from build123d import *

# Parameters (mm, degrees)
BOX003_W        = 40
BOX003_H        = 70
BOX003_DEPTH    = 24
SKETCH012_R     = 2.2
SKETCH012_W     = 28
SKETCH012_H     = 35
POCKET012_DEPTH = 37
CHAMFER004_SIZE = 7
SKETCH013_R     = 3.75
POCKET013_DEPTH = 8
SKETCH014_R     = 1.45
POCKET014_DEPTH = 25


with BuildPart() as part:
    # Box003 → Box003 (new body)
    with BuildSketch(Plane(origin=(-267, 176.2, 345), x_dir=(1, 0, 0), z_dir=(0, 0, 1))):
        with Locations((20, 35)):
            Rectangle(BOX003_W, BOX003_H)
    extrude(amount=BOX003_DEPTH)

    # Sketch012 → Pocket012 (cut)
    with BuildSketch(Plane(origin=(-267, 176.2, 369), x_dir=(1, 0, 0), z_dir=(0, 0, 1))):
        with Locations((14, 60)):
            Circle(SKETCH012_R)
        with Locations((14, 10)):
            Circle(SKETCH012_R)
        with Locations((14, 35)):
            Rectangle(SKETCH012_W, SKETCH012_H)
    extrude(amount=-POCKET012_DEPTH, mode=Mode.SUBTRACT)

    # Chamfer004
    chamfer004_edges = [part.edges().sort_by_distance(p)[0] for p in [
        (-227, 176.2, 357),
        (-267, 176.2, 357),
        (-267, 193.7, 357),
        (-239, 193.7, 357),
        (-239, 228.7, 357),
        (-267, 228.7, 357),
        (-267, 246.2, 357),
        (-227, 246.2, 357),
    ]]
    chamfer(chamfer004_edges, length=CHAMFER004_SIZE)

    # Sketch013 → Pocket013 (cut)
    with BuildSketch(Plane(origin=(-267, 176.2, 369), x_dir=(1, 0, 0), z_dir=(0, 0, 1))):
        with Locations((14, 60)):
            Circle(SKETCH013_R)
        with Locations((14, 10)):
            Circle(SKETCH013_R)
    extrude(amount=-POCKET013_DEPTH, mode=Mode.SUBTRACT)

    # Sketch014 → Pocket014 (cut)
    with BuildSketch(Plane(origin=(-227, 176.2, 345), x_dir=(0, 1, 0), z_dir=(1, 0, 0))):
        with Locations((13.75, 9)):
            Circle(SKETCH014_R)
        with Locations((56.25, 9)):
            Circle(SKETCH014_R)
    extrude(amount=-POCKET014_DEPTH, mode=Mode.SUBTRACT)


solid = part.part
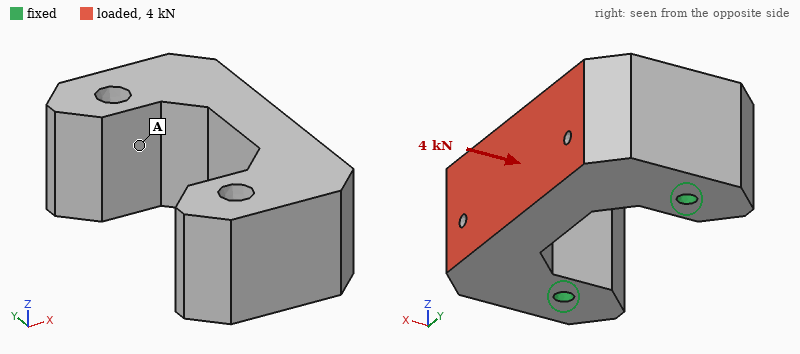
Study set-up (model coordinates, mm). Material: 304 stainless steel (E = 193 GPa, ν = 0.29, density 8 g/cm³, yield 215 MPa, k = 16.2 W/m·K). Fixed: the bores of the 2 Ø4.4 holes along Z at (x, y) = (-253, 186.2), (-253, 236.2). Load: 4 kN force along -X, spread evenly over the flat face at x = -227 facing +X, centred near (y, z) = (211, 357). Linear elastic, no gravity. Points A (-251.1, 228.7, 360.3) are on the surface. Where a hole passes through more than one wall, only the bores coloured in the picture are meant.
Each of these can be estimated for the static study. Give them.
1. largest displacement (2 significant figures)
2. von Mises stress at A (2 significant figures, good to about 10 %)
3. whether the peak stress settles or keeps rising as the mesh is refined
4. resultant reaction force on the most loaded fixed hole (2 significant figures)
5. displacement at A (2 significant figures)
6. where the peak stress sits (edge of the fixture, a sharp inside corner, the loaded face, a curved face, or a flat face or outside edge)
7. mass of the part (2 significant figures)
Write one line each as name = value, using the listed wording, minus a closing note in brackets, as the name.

largest displacement = 3.2 µm
von Mises stress at A = 6.7 MPa
whether the peak stress settles or keeps rising as the mesh is refined = keeps rising
resultant reaction force on the most loaded fixed hole = 2.2 kN
displacement at A = 0.57 µm
where the peak stress sits = edge of the fixture
mass of the part = 320 g
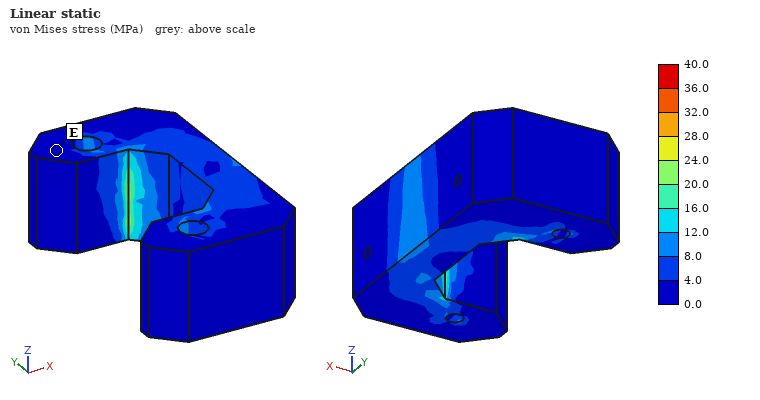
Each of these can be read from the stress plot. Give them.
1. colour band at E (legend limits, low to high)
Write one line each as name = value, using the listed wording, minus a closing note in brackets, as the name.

colour band at E = 0.0 to 4.0 MPa
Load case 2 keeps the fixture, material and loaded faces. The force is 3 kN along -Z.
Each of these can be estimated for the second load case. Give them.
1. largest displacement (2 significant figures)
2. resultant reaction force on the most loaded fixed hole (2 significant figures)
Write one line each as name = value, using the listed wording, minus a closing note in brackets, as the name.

largest displacement = 10 µm
resultant reaction force on the most loaded fixed hole = 1.5 kN
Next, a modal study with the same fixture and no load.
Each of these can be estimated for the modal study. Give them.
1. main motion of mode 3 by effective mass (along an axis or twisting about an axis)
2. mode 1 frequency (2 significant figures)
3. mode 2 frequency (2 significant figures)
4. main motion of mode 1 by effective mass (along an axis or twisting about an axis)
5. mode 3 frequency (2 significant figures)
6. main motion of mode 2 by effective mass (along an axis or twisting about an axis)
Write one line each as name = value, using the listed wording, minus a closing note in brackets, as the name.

main motion of mode 3 by effective mass = twisting about X
mode 1 frequency = 9100 Hz
mode 2 frequency = 12 kHz
main motion of mode 1 by effective mass = along Z
mode 3 frequency = 14 kHz
main motion of mode 2 by effective mass = along Y
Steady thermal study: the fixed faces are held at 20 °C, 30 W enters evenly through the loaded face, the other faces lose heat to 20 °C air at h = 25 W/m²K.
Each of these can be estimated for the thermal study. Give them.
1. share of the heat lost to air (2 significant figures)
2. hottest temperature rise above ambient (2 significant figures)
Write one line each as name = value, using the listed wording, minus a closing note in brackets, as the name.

share of the heat lost to air = 17 %
hottest temperature rise above ambient = 64 K
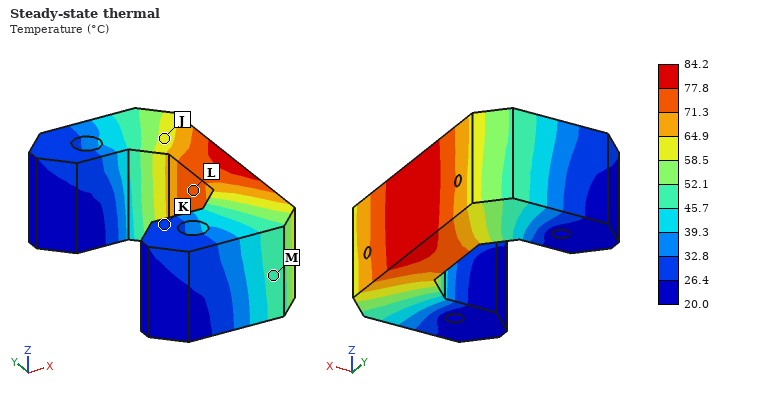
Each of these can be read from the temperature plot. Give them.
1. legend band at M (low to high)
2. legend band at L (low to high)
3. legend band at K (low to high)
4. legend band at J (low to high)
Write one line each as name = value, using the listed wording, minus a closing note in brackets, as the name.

legend band at M = 45.7 to 52.1 °C
legend band at L = 71.3 to 77.8 °C
legend band at K = 26.4 to 32.8 °C
legend band at J = 58.5 to 64.9 °C
